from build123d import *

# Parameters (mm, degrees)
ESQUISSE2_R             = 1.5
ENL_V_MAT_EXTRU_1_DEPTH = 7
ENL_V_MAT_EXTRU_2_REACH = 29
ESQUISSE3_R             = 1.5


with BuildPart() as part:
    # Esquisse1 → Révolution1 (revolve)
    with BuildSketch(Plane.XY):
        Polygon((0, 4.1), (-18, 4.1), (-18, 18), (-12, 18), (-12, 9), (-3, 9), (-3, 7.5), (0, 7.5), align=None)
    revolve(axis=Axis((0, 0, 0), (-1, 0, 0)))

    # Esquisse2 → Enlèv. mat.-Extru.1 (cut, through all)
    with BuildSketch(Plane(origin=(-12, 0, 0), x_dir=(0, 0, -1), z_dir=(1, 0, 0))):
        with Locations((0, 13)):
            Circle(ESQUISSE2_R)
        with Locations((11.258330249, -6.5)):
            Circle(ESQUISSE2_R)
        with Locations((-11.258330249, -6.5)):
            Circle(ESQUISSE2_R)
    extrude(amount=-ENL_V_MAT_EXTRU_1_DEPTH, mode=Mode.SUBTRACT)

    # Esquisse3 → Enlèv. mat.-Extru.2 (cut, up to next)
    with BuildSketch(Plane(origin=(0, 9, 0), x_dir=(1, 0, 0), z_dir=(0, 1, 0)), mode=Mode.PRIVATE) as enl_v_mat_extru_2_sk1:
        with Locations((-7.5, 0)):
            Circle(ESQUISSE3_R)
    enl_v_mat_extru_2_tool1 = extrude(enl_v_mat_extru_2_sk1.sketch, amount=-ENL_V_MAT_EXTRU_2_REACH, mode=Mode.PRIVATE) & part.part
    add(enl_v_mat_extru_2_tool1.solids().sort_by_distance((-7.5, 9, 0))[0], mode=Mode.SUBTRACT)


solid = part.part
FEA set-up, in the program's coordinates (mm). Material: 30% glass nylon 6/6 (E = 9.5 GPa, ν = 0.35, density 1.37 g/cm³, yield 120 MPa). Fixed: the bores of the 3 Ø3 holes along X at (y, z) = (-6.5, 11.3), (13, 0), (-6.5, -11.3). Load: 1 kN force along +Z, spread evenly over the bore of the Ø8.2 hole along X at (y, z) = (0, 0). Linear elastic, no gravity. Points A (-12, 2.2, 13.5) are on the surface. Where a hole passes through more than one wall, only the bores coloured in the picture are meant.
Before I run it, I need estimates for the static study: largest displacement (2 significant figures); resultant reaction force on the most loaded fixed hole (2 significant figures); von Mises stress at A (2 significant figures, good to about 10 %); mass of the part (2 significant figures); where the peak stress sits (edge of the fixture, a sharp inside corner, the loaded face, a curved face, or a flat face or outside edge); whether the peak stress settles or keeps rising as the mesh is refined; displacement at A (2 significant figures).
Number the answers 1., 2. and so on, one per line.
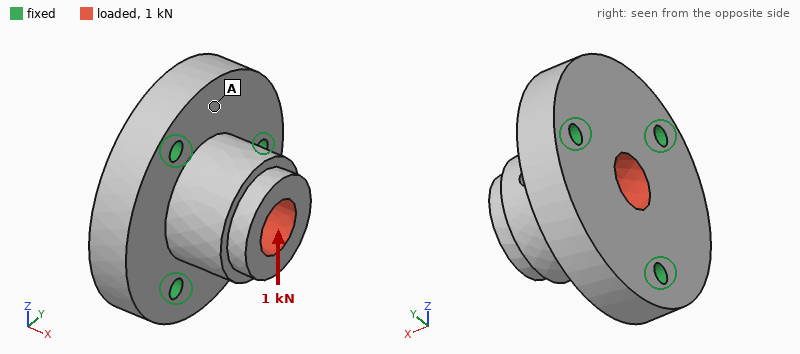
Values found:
1. 34 µm
2. 430 N
3. 2.5 MPa
4. 11 g
5. edge of the fixture
6. keeps rising
7. 10 µm
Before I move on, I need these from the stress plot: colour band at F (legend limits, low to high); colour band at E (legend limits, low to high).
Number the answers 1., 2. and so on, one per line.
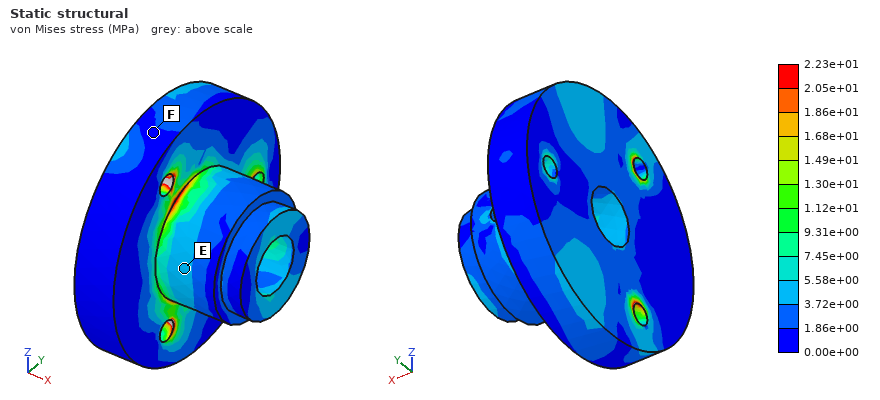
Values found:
1. 0.00e+00 to 1.86e+00 MPa
2. 3.72e+00 to 5.58e+00 MPa
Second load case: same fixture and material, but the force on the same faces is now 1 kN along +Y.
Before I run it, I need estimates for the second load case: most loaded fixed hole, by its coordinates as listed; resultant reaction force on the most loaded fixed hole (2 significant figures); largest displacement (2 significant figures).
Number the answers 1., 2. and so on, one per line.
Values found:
1. (13, 0)
2. 470 N
3. 35 µm
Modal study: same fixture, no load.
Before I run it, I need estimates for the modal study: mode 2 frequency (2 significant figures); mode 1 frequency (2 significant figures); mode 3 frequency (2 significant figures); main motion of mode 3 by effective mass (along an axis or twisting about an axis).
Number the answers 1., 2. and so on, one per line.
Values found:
1. 13 kHz
2. 13 kHz
3. 16 kHz
4. along X
